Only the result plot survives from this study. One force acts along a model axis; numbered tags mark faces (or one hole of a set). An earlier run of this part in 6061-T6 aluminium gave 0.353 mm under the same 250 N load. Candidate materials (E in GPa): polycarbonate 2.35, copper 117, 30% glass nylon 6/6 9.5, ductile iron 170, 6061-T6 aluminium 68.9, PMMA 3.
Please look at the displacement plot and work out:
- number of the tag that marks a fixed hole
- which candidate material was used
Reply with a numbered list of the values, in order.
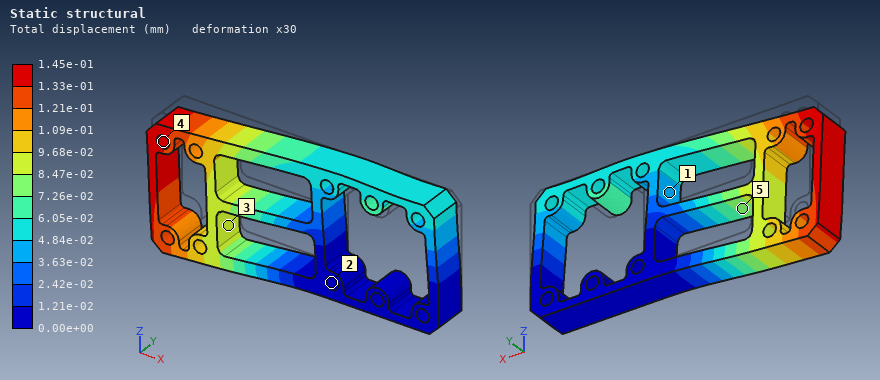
1. 2
2. ductile iron
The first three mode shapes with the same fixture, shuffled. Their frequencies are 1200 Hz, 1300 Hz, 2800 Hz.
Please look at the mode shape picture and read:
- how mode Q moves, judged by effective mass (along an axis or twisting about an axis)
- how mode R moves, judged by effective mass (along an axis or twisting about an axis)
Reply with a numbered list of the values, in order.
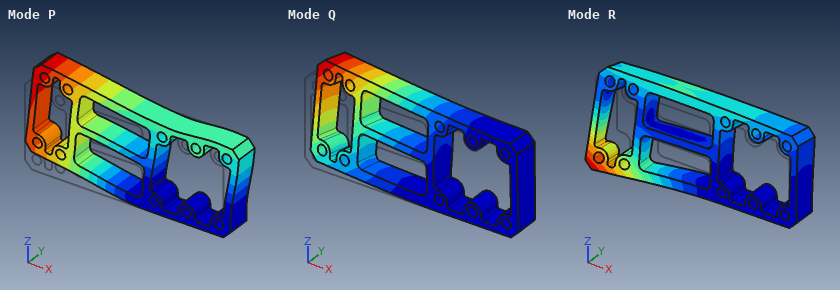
1. along Y
2. twisting about X
